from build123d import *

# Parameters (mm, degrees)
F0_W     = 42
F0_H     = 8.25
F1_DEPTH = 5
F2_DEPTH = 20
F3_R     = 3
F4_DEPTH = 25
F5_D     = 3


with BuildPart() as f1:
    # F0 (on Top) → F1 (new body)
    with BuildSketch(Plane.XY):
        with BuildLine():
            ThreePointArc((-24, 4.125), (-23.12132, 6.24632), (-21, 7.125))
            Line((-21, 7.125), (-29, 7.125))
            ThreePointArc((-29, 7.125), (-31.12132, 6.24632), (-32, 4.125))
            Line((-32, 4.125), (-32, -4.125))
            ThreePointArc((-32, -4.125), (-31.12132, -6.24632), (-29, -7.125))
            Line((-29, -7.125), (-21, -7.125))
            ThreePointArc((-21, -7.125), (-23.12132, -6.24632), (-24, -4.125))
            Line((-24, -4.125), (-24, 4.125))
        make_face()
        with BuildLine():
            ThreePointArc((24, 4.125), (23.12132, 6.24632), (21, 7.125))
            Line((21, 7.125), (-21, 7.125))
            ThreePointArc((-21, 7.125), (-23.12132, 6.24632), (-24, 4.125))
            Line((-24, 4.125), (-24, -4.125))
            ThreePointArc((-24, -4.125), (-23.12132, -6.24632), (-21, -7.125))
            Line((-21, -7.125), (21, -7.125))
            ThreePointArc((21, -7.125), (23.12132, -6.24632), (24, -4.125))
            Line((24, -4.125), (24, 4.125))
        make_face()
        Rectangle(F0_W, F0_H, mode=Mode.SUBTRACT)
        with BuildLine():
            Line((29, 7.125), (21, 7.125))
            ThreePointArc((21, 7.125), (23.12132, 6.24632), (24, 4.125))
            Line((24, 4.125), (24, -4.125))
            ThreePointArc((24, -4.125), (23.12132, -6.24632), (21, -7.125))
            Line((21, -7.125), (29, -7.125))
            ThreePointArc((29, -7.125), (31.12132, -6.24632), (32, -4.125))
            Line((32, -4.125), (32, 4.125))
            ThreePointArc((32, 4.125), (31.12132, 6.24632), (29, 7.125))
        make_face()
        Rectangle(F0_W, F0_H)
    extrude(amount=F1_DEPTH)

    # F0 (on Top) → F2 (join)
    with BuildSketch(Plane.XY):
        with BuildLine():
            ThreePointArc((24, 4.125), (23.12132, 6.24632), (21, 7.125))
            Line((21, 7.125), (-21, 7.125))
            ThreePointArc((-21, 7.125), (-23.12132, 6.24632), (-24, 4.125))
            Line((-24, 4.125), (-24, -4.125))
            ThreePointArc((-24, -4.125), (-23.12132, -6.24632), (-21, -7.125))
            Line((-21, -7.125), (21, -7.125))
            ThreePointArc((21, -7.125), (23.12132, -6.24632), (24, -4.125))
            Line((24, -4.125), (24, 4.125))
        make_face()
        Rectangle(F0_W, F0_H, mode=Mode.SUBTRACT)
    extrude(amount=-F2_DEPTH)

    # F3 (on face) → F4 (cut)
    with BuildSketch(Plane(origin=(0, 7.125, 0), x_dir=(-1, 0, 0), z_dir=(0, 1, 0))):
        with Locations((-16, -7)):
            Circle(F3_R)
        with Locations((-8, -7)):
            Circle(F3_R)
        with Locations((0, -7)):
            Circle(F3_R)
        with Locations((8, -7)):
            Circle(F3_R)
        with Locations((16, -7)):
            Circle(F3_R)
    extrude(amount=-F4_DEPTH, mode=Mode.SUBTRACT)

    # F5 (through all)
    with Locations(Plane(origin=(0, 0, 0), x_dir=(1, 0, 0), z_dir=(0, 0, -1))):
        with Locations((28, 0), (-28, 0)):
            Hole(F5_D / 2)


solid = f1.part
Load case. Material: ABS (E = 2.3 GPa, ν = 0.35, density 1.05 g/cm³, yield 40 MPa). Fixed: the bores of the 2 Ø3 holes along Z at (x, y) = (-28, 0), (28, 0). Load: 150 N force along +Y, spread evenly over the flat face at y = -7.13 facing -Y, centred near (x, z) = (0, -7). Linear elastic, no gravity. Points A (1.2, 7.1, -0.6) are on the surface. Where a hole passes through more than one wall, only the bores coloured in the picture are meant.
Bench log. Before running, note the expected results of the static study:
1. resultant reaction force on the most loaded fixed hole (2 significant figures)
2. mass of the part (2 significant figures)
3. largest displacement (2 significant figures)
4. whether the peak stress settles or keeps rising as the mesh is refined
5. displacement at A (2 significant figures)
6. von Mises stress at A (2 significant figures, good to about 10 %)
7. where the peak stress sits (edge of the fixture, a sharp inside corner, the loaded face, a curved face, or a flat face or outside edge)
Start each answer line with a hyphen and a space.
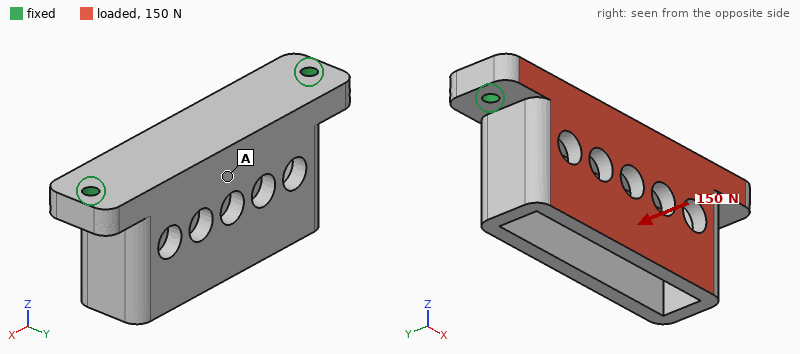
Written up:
- 75 N
- 11 g
- 0.60 mm
- keeps rising
- 0.13 mm
- 2.4 MPa
- edge of the fixture
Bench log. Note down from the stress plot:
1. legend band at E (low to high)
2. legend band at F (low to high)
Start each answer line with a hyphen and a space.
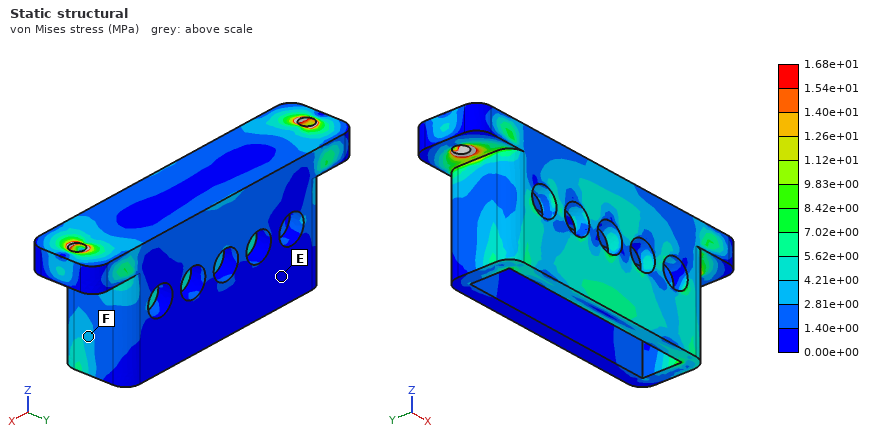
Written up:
- 0.00e+00 to 1.40e+00 MPa
- 2.81e+00 to 4.21e+00 MPa
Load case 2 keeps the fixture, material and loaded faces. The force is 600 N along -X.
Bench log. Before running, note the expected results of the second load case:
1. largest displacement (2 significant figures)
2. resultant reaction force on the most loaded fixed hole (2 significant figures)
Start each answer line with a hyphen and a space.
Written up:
- 0.17 mm
- 330 N
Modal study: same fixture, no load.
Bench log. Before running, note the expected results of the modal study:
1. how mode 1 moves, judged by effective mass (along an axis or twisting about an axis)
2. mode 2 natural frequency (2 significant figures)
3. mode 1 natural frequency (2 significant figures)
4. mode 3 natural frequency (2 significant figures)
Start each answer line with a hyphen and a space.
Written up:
- along Y
- 2500 Hz
- 1300 Hz
- 2600 Hz
